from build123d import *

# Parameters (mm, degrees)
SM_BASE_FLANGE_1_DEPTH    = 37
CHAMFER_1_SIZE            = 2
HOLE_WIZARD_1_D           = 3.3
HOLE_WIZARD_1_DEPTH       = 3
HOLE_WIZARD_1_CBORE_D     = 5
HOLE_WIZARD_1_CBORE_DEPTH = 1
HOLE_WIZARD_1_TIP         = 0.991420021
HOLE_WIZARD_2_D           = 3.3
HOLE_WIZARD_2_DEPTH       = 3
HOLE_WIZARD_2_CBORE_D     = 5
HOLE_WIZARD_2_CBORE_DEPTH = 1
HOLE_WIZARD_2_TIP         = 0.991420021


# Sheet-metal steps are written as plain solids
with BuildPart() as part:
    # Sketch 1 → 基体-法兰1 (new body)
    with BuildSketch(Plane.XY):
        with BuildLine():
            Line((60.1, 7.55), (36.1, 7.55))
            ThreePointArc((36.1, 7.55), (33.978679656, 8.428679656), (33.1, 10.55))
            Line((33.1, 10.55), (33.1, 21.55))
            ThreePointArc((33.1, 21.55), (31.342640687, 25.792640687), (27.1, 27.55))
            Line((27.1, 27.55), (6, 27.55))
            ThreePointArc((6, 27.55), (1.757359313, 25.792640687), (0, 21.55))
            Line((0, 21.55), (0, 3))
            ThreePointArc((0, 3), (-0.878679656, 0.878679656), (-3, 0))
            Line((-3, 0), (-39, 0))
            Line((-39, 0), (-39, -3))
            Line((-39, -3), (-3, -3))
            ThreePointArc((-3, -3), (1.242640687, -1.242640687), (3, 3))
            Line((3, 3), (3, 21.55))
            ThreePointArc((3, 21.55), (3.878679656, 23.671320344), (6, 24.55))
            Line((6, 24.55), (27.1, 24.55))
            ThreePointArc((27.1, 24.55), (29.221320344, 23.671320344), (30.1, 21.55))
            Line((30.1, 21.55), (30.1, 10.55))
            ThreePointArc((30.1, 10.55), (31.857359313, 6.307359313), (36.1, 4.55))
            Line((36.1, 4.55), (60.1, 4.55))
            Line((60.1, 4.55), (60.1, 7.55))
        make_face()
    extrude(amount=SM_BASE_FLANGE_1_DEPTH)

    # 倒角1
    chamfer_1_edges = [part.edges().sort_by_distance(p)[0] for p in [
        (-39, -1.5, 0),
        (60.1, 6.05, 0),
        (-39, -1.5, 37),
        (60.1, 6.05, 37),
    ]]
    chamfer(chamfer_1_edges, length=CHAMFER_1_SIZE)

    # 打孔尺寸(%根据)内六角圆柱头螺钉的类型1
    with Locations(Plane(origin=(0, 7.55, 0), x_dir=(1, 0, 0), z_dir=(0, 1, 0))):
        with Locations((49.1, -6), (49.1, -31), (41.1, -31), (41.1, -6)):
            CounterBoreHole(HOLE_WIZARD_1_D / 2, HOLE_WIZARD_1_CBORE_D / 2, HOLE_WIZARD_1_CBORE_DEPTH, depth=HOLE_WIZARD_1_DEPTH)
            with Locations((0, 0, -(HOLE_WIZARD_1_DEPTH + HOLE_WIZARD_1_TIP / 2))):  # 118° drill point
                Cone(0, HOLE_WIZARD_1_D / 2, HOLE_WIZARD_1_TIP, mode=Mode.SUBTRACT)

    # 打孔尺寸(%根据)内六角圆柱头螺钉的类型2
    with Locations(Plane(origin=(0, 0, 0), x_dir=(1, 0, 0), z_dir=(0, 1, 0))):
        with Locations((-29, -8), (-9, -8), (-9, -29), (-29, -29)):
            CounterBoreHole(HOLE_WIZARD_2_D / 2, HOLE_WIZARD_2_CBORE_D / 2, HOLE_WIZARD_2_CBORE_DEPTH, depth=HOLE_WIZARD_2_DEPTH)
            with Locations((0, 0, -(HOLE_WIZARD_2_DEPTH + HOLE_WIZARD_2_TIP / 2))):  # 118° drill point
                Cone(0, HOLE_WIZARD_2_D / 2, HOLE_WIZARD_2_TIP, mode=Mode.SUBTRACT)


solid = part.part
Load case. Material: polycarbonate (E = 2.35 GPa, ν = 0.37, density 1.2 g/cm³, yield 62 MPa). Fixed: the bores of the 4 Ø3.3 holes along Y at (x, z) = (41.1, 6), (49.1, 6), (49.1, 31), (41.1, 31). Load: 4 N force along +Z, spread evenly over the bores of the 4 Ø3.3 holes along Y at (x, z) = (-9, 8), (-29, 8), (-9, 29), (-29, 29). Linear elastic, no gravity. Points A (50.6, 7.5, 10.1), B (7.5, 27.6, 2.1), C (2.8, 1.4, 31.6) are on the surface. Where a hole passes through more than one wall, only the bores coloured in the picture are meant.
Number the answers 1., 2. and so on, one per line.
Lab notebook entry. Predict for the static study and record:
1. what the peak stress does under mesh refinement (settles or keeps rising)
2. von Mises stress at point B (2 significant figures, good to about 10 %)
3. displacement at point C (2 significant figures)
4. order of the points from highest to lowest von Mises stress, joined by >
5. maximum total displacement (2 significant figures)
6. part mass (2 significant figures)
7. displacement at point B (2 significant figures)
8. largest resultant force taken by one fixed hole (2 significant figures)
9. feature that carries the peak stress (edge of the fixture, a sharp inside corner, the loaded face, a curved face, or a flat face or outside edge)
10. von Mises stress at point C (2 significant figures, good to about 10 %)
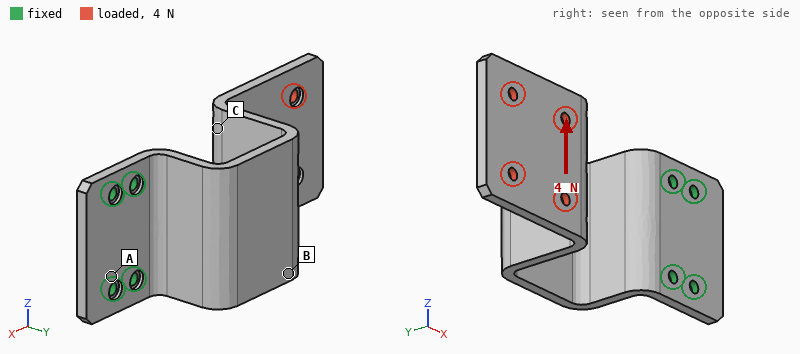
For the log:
1. keeps rising
2. 1.4 MPa
3. 0.62 mm
4. B > C > A
5. 1.2 mm
6. 18 g
7. 0.33 mm
8. 6.2 N
9. edge of the fixture
10. 0.66 MPa
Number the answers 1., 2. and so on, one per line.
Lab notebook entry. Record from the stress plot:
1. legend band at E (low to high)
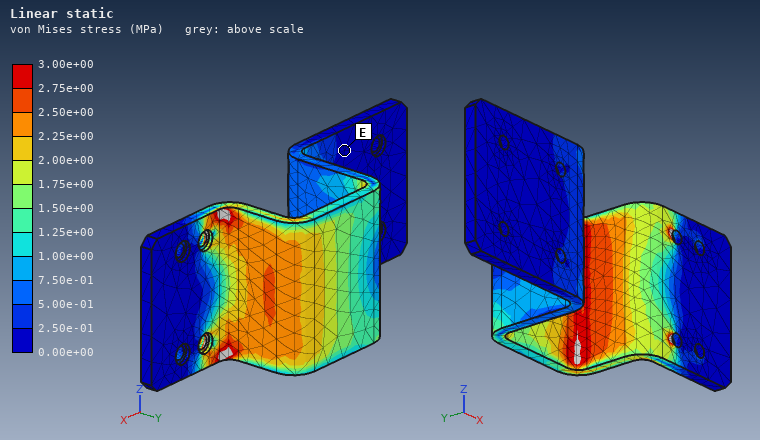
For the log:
1. 0.00e+00 to 2.50e-01 MPa
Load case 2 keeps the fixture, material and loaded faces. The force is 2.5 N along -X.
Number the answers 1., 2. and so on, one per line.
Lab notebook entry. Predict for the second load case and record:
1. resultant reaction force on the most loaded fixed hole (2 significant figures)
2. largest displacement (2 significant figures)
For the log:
1. 1.6 N
2. 1.1 mm
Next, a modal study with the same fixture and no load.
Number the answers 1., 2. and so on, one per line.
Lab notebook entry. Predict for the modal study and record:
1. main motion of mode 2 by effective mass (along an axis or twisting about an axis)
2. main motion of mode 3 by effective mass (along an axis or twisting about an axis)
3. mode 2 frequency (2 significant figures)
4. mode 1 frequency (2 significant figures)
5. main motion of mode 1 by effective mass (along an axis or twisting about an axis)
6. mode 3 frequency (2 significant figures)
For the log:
1. along Z
2. along X
3. 130 Hz
4. 73 Hz
5. along Y
6. 240 Hz
